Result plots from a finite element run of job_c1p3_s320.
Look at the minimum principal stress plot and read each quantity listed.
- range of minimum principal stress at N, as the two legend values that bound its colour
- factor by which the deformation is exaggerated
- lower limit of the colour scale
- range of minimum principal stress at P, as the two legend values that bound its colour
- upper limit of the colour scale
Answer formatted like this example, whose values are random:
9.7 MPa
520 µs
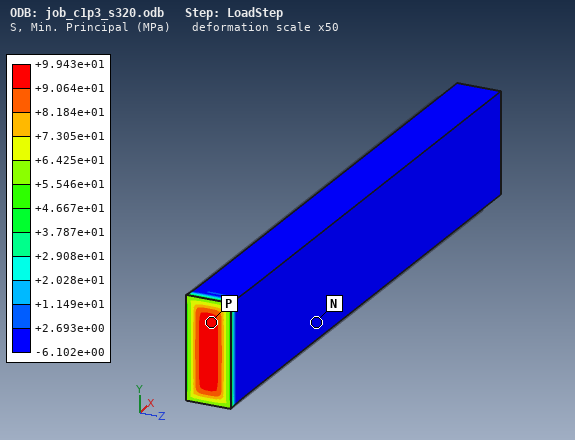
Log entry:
-6.102e+00 to +2.693e+00 MPa
50
-6.102e+00 MPa
+9.064e+01 to +9.943e+01 MPa
+9.943e+01 MPa
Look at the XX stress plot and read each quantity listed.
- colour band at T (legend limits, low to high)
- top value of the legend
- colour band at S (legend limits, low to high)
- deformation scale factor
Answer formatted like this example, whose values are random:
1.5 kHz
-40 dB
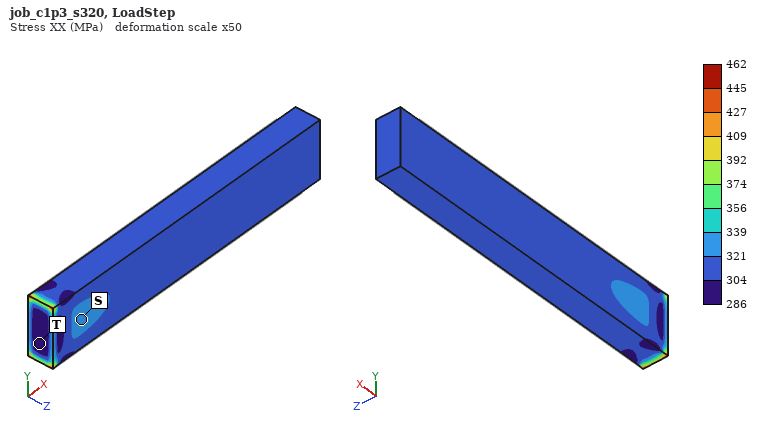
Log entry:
286 to 304 MPa
462 MPa
321 to 339 MPa
50
